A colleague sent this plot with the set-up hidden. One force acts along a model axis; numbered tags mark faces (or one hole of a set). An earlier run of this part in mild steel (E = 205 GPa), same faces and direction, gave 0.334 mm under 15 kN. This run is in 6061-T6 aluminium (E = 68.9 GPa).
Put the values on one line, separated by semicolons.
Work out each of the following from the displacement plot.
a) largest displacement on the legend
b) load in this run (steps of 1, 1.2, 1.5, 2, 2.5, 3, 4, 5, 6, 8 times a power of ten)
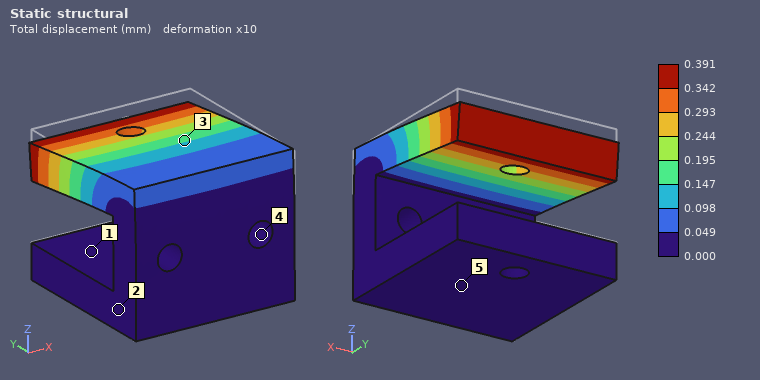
0.391 mm; 6 kN
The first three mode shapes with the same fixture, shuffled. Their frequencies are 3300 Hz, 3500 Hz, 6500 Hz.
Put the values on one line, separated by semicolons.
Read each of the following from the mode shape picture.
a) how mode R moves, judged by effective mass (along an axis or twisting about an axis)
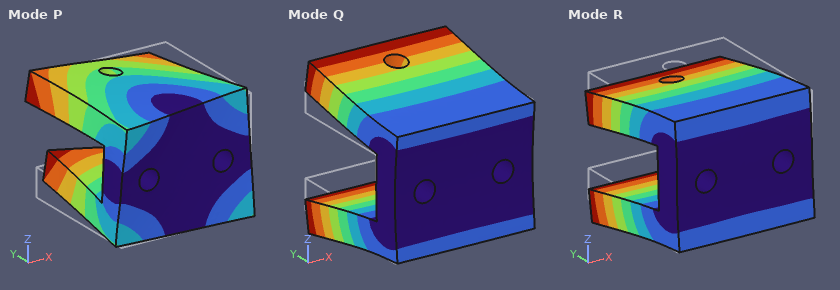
along Z
